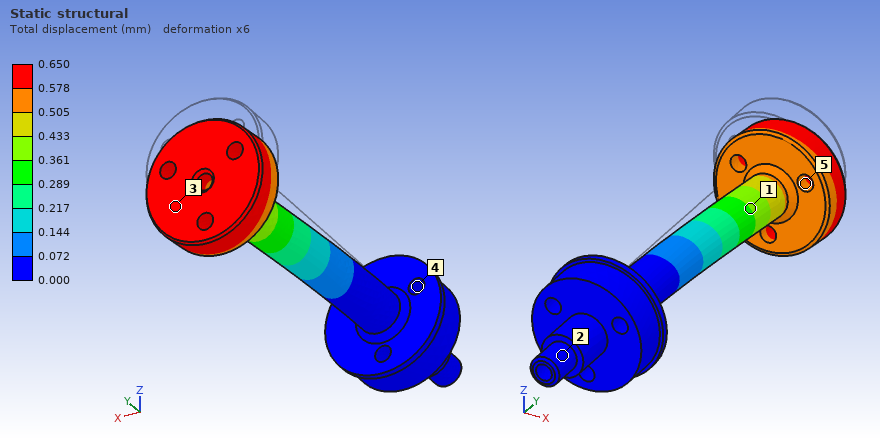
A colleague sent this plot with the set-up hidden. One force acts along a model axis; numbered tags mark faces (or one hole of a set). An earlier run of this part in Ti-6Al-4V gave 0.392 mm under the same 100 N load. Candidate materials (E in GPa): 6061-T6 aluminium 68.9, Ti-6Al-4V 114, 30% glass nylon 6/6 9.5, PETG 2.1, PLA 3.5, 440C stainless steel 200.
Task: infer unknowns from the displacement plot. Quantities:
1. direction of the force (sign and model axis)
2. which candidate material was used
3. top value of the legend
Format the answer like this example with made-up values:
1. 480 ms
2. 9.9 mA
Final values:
1. -Z
2. 6061-T6 aluminium
3. 0.650 mm
